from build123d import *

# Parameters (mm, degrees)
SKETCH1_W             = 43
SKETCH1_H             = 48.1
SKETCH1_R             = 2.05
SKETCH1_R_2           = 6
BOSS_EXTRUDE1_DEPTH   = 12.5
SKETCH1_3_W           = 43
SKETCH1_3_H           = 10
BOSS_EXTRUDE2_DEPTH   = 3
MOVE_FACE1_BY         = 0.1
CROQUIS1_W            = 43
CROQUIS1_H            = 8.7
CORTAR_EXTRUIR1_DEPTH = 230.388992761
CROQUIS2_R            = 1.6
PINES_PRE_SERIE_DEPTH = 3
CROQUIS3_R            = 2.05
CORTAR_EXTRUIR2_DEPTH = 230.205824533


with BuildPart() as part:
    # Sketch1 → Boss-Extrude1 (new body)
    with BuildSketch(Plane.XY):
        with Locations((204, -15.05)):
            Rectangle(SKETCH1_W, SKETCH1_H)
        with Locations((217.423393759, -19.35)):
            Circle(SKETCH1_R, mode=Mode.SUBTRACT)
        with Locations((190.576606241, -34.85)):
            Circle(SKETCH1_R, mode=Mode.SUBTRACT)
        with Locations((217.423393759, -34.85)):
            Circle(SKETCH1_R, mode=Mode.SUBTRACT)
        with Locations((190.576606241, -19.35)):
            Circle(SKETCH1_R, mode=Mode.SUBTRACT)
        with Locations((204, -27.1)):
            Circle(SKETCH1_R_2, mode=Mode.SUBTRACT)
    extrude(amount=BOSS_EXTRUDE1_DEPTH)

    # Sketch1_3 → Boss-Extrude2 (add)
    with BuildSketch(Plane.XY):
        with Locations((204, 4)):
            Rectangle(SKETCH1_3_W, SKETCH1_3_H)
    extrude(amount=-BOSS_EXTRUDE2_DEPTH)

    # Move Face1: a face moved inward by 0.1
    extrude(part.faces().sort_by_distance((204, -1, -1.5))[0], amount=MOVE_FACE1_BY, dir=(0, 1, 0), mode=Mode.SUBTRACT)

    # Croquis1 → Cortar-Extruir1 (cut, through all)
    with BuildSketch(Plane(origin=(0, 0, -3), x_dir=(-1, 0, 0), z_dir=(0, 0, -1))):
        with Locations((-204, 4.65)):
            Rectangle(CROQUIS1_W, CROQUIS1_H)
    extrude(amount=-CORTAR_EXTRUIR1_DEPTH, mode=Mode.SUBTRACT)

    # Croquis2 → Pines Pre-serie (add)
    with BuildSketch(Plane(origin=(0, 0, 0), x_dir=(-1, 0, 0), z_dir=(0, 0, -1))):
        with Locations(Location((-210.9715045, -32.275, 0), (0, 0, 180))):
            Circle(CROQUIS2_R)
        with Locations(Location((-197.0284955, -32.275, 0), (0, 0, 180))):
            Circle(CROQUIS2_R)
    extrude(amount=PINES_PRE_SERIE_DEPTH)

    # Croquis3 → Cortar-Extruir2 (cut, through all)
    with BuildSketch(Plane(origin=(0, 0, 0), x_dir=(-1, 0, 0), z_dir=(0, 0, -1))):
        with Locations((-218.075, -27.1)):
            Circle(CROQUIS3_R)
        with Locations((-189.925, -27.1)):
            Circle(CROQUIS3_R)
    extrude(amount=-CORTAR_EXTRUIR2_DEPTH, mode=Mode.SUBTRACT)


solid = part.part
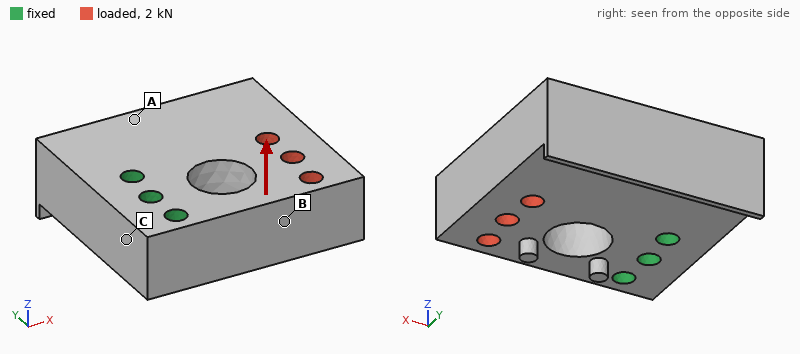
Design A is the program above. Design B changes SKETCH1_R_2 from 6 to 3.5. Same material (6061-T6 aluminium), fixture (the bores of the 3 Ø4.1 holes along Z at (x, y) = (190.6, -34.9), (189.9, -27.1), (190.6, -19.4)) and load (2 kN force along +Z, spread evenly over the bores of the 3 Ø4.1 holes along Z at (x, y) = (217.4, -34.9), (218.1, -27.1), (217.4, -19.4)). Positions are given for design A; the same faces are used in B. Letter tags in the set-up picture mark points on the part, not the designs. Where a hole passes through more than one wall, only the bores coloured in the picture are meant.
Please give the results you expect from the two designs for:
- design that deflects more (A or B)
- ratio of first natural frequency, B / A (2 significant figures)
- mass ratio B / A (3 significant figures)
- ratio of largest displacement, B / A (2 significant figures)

A
1.1
1.05
0.81
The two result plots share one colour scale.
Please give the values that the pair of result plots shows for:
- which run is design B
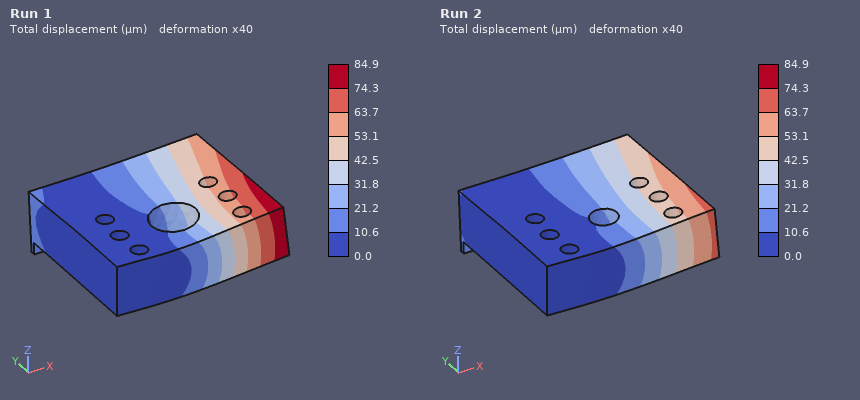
Run 2
